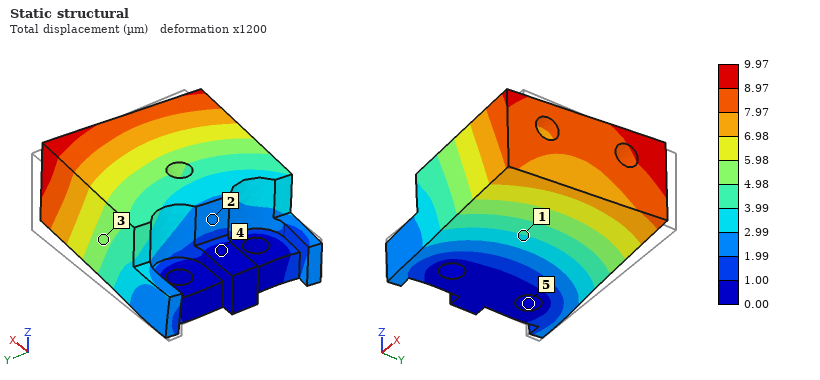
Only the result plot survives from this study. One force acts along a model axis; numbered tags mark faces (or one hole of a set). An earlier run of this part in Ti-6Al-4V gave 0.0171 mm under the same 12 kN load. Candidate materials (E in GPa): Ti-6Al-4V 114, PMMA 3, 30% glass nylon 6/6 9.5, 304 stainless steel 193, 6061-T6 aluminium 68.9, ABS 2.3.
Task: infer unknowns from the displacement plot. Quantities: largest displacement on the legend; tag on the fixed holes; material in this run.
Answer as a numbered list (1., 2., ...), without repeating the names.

1. 9.97 µm
2. 5
3. 304 stainless steel
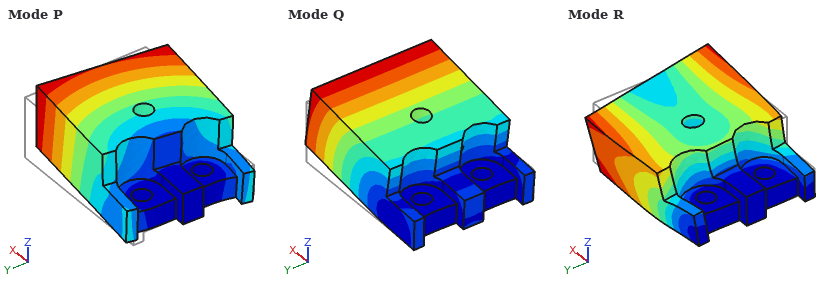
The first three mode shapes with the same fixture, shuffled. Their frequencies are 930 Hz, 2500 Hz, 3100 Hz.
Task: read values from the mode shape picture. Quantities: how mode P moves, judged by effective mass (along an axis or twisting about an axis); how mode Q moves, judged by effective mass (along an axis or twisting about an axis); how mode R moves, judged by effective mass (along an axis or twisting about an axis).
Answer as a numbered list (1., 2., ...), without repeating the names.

1. along Y
2. along Z
3. twisting about X
